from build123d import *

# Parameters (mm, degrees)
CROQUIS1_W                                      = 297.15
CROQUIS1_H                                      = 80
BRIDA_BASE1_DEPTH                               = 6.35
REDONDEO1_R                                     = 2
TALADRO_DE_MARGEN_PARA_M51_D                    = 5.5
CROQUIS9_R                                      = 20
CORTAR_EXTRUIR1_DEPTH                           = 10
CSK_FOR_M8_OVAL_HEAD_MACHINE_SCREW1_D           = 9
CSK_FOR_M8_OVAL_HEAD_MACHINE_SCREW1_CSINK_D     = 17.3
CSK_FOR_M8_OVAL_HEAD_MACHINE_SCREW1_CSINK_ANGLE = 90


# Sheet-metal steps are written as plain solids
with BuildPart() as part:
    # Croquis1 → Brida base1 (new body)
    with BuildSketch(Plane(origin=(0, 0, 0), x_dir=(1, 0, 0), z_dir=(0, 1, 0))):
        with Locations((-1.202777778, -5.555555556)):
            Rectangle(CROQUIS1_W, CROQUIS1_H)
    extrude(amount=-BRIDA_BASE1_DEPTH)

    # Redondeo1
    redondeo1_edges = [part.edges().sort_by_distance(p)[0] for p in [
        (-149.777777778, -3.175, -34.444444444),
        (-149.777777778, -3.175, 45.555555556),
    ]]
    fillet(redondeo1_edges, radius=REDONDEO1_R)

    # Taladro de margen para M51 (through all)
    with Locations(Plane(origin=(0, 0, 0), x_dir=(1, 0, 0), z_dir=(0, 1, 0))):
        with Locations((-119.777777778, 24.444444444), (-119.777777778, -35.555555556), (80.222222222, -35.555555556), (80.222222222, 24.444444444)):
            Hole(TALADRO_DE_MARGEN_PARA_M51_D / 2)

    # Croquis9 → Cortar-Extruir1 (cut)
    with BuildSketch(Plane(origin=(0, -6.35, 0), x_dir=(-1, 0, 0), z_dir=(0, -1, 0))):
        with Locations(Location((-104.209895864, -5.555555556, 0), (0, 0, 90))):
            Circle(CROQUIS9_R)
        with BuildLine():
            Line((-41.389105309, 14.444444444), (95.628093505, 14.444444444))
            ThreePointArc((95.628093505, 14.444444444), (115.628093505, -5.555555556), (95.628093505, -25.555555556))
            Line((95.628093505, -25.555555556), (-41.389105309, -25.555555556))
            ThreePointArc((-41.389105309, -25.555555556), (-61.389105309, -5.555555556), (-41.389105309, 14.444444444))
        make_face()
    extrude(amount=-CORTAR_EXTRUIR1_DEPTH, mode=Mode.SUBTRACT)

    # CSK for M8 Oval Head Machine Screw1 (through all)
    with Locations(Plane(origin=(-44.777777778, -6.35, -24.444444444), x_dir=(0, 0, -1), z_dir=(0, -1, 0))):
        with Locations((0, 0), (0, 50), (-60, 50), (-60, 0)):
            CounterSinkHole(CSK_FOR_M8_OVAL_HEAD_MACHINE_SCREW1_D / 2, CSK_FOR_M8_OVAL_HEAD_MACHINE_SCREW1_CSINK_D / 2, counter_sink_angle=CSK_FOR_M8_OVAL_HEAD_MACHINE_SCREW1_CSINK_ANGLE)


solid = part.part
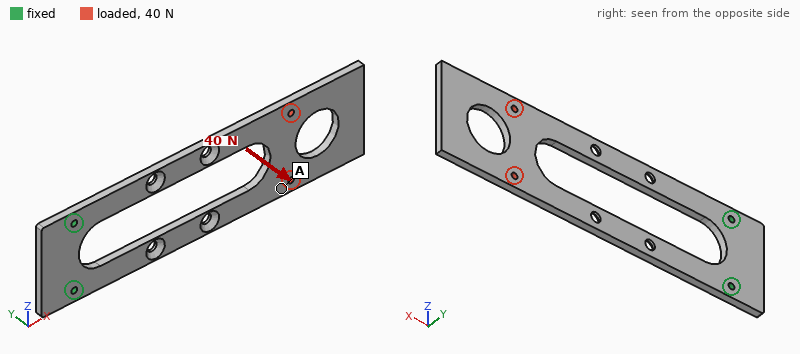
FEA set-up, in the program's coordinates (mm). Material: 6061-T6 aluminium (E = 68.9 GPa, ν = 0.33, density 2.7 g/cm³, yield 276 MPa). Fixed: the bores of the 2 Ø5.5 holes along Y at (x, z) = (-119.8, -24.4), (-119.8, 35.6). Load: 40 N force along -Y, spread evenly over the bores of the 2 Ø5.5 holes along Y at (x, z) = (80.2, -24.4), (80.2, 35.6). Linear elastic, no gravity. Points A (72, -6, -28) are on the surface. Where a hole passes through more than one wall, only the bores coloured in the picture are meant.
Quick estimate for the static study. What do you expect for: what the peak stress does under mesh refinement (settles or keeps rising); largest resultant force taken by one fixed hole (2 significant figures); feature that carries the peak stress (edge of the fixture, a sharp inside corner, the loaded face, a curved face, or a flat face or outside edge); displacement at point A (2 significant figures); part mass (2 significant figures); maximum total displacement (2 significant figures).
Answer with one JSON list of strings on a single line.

["keeps rising", "20 N", "a sharp inside corner", "1.9 mm", "260 g", "3.1 mm"]
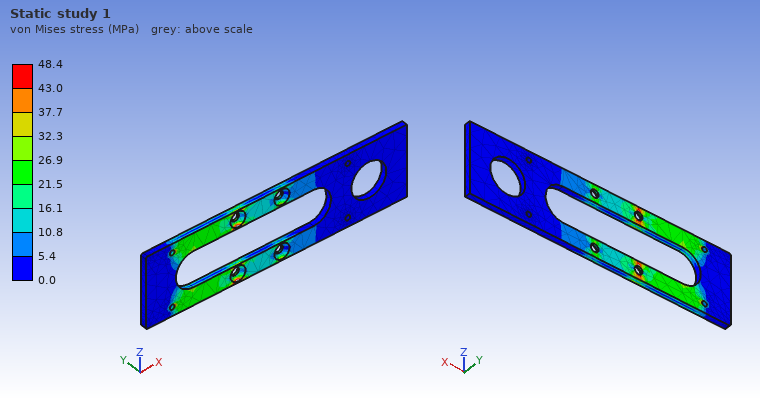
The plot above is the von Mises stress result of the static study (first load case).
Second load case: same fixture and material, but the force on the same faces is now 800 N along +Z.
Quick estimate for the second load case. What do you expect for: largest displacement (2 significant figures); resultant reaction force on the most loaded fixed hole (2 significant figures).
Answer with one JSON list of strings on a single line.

["0.90 mm", "2.5 kN"]
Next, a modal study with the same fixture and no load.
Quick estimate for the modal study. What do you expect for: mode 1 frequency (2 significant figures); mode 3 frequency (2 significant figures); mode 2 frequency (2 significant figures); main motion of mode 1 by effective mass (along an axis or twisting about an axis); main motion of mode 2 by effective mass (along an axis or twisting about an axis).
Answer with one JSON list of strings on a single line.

["55 Hz", "410 Hz", "320 Hz", "along Y", "twisting about X"]
